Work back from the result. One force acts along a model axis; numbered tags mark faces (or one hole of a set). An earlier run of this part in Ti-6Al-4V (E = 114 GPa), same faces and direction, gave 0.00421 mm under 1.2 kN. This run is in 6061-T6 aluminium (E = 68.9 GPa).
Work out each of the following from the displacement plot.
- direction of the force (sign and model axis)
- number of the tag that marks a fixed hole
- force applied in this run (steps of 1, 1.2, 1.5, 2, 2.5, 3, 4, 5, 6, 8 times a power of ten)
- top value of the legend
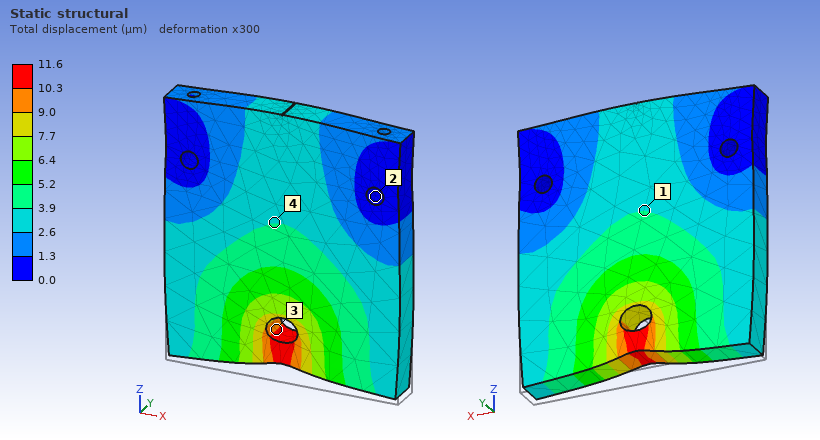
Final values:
+Z
2
2 kN
11.6 µm
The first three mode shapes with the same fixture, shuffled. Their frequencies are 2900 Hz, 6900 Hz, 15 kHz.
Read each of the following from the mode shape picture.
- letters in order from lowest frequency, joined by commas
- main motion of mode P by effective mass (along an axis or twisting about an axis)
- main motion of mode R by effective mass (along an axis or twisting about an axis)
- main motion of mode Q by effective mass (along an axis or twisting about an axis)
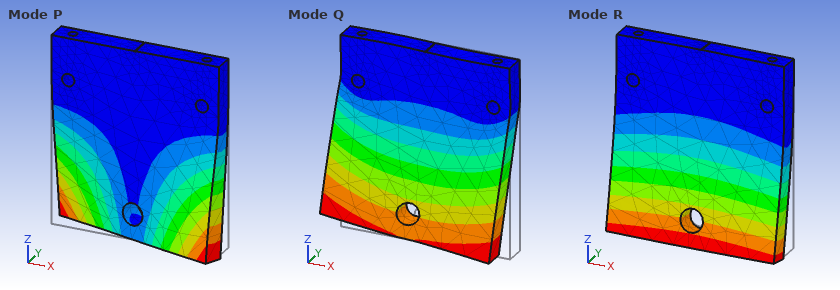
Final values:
R, P, Q
twisting about Z
along Y
along X
